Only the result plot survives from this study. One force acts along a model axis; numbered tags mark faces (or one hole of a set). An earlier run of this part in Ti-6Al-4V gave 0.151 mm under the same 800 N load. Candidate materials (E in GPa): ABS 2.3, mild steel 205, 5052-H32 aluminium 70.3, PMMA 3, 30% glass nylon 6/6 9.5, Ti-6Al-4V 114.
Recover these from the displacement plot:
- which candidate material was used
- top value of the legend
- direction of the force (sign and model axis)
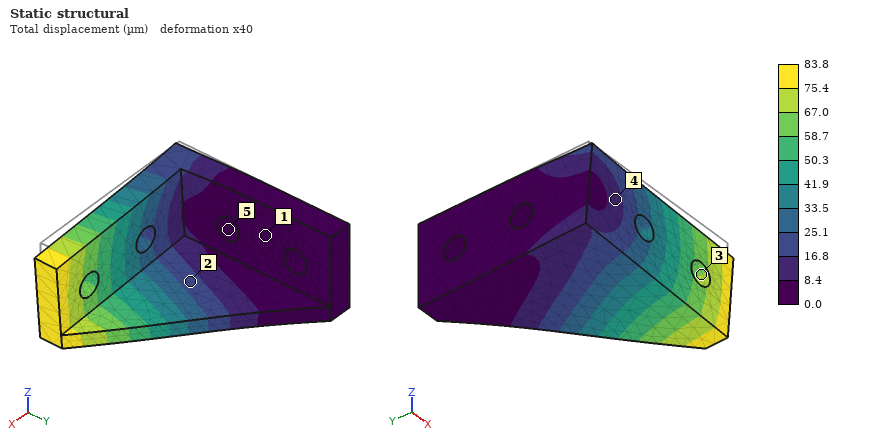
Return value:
mild steel
83.8 µm
-Z
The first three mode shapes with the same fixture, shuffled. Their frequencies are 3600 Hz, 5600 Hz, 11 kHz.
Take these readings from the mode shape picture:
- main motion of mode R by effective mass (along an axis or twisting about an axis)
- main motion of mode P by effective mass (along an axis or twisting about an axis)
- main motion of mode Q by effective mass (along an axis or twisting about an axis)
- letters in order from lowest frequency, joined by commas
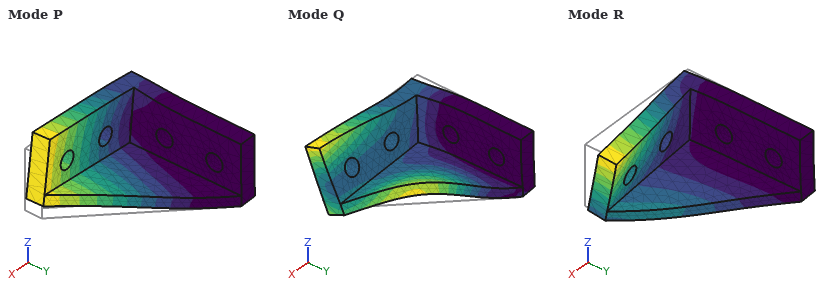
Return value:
along Y
along Z
along X
P, R, Q
